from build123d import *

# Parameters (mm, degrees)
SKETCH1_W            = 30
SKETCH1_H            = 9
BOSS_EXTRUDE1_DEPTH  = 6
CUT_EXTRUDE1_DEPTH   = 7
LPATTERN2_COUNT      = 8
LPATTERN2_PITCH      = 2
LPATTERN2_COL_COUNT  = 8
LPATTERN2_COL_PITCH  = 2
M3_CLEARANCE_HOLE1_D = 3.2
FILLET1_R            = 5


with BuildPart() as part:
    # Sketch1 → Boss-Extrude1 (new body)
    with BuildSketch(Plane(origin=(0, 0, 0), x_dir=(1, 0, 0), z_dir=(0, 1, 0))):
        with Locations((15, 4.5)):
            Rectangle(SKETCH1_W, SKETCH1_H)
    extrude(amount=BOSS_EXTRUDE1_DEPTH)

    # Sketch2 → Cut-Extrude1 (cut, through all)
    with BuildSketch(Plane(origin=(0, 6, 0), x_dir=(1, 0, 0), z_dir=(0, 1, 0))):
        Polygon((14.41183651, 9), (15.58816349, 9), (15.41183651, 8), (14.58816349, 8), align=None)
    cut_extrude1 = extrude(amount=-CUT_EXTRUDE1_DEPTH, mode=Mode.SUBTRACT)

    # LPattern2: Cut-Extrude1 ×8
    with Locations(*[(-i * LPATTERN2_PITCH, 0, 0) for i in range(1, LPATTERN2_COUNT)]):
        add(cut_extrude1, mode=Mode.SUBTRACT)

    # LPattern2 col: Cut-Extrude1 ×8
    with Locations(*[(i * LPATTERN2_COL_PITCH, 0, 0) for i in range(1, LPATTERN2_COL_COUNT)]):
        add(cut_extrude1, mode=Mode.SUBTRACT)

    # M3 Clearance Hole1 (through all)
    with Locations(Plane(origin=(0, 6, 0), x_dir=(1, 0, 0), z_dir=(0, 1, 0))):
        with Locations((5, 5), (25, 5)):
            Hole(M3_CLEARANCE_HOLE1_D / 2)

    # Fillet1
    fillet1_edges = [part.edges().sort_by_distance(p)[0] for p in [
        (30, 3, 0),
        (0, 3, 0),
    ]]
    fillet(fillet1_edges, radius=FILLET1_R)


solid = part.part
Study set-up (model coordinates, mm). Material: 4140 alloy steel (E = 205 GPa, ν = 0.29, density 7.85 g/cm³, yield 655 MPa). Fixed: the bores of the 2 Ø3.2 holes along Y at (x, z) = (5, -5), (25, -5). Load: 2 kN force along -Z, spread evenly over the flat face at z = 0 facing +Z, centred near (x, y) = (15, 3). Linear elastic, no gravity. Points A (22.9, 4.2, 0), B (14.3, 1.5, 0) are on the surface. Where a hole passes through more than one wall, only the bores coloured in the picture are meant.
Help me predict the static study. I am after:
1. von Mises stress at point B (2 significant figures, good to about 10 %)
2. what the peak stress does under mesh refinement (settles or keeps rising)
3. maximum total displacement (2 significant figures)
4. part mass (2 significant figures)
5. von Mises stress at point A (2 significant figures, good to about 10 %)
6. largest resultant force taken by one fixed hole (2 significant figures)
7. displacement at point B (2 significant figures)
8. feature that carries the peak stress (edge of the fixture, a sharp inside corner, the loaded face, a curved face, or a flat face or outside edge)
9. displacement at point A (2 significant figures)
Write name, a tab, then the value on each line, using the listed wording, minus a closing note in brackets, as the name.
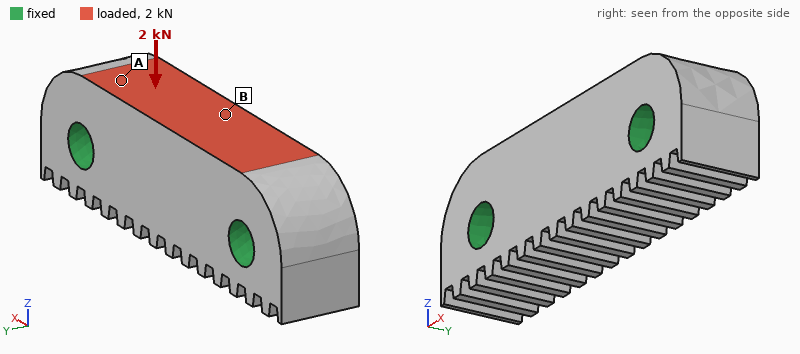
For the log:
von Mises stress at point B	37 MPa
what the peak stress does under mesh refinement	keeps rising
maximum total displacement	2.5 µm
part mass	11 g
von Mises stress at point A	19 MPa
largest resultant force taken by one fixed hole	1.0 kN
displacement at point B	2.4 µm
feature that carries the peak stress	edge of the fixture
displacement at point A	1.2 µm
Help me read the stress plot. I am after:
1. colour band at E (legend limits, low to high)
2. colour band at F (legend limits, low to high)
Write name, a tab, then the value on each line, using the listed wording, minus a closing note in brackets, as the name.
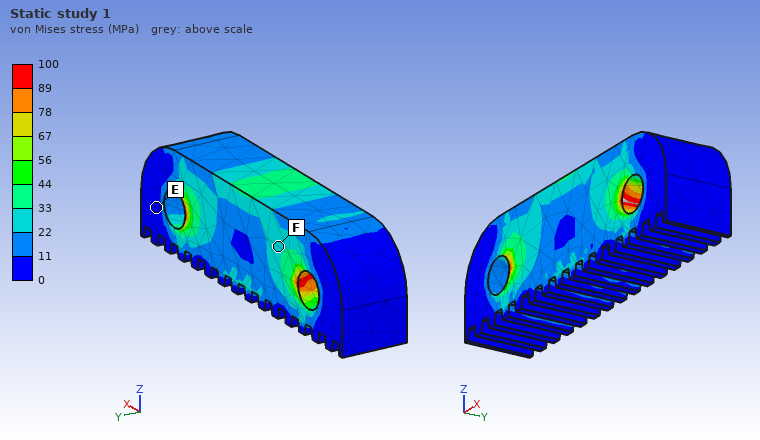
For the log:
colour band at E	0 to 11 MPa
colour band at F	22 to 33 MPa
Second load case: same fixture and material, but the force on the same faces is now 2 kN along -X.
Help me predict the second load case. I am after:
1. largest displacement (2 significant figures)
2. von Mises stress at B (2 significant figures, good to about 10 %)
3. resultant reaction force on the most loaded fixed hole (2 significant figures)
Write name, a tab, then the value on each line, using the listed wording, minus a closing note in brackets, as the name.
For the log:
largest displacement	1.2 µm
von Mises stress at B	29 MPa
resultant reaction force on the most loaded fixed hole	1.1 kN
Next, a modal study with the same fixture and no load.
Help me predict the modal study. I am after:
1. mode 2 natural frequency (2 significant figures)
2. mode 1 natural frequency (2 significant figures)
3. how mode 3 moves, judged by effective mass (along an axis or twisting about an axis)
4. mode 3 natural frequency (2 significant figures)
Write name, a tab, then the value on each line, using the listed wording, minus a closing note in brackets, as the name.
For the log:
mode 2 natural frequency	57 kHz
mode 1 natural frequency	57 kHz
how mode 3 moves, judged by effective mass	twisting about X
mode 3 natural frequency	70 kHz
